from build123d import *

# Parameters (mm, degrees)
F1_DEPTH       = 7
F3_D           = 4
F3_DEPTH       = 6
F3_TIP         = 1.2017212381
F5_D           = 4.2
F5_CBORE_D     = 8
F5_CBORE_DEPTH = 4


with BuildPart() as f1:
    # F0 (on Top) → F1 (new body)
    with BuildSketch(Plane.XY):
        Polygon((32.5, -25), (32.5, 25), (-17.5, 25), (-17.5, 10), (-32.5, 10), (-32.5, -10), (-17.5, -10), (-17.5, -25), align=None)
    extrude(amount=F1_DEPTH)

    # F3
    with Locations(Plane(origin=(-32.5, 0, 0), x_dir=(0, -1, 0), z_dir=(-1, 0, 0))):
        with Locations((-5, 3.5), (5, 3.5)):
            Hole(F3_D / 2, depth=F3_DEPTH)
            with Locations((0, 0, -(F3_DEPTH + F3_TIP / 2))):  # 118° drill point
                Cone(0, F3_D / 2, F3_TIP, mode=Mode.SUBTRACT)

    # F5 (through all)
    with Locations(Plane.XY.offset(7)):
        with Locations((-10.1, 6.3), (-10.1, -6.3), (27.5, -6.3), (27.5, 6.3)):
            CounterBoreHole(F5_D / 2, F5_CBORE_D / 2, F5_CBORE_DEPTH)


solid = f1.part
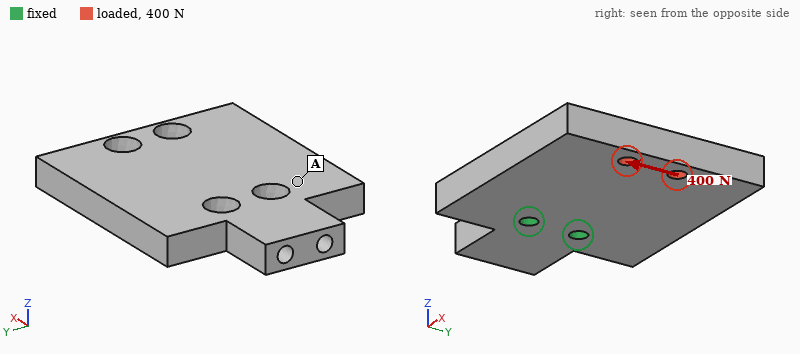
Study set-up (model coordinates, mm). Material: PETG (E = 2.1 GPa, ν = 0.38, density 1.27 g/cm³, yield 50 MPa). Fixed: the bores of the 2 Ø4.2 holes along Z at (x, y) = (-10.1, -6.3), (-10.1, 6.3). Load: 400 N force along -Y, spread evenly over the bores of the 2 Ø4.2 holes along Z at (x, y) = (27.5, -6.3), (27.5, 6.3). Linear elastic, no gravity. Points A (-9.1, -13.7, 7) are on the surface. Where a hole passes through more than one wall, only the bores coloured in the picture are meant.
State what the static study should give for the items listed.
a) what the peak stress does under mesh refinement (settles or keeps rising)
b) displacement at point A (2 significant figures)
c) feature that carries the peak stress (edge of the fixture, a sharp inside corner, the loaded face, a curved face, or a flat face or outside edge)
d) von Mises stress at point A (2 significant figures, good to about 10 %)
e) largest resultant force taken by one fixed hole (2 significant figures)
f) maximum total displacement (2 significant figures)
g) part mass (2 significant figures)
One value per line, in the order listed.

keeps rising
0.16 mm
edge of the fixture
6.4 MPa
980 N
0.78 mm
23 g
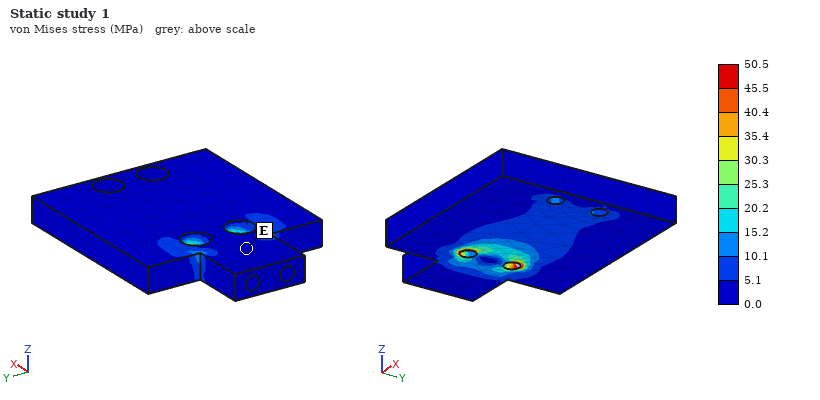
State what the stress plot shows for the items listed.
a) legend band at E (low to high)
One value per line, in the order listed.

0.0 to 5.1 MPa
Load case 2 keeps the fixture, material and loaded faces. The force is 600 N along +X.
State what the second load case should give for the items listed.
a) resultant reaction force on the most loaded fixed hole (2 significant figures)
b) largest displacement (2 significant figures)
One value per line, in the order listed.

300 N
0.35 mm
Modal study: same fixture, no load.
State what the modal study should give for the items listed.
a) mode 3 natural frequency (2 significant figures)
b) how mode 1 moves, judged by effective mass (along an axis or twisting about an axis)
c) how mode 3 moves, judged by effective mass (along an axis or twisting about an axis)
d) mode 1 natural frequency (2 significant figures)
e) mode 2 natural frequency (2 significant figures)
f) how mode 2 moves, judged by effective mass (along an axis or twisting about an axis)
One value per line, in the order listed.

1400 Hz
along Z
along Y
480 Hz
1100 Hz
twisting about X
